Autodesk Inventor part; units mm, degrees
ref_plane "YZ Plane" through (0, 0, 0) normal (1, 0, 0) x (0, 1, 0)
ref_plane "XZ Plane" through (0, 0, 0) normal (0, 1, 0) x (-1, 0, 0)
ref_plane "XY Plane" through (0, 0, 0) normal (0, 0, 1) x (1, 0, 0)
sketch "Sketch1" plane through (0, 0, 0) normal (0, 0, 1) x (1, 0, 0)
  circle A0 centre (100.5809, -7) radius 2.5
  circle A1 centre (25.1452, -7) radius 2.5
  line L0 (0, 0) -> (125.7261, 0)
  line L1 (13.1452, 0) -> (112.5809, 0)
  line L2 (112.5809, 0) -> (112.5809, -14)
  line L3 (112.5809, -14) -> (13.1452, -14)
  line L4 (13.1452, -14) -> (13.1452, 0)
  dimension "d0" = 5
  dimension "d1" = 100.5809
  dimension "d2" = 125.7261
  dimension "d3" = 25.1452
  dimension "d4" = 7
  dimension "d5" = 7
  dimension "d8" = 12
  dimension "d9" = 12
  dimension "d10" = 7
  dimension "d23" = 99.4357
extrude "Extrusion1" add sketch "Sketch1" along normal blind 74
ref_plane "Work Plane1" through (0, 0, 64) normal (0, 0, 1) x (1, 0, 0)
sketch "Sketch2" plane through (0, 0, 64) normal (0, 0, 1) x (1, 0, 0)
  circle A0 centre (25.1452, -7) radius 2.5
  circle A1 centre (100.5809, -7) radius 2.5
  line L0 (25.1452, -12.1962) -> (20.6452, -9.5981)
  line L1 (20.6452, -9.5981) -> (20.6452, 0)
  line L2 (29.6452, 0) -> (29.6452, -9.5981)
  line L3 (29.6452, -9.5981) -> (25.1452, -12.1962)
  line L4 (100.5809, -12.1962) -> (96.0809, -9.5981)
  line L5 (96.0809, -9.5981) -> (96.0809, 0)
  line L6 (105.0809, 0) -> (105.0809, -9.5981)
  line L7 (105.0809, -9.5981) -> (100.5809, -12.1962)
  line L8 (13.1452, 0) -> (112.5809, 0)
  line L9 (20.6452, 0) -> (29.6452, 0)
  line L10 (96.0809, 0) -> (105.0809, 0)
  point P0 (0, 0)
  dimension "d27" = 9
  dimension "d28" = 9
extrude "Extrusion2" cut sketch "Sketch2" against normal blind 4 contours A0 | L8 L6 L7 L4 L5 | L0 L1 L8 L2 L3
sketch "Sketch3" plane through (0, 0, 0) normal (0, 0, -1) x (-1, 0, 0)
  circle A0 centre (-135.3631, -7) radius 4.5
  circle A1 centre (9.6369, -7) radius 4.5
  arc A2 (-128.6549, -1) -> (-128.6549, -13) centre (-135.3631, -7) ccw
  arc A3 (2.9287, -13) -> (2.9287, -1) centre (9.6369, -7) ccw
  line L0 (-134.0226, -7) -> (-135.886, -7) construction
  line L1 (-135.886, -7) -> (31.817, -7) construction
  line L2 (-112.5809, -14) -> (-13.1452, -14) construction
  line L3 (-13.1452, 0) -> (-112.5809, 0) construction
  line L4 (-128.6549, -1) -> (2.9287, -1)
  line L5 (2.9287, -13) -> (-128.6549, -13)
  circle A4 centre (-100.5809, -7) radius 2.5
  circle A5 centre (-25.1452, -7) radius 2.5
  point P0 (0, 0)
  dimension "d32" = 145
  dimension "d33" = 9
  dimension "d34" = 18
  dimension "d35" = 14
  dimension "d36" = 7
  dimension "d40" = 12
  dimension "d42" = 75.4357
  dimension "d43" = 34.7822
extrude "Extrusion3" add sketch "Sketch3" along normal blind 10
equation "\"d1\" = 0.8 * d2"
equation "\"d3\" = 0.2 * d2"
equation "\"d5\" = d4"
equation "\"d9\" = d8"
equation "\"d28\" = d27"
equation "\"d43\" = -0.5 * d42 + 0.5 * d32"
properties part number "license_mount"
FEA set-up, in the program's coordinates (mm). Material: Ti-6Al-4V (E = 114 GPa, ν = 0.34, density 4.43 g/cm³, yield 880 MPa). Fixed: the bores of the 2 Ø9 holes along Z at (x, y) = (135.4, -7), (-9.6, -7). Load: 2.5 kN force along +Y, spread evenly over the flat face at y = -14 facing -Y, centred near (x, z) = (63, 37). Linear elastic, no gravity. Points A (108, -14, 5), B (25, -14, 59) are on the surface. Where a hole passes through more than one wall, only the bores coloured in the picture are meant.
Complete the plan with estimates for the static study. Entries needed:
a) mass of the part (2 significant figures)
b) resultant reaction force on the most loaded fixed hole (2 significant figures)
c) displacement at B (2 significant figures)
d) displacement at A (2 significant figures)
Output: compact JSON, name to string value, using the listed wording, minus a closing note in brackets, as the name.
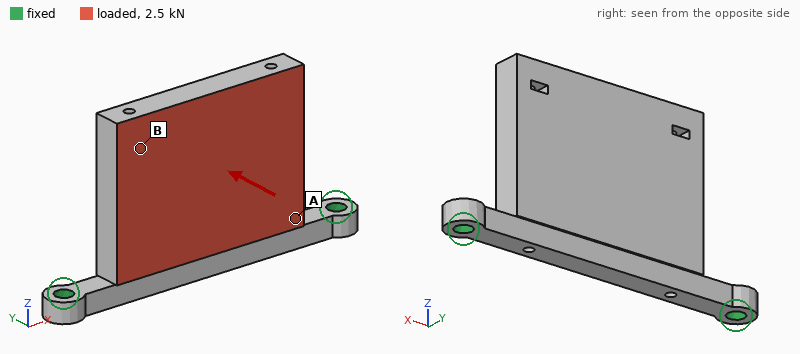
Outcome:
{"mass of the part": "520 g", "resultant reaction force on the most loaded fixed hole": "1.3 kN", "displacement at B": "1.0 mm", "displacement at A": "0.19 mm"}
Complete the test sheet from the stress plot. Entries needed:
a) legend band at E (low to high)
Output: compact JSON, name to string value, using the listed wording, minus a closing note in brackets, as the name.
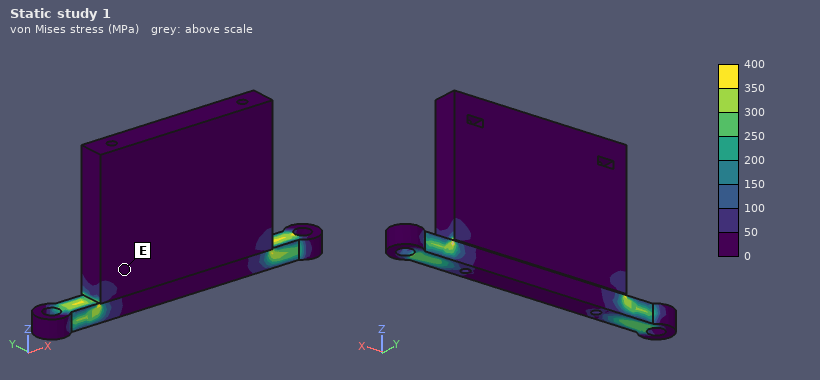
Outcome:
{"legend band at E": "0 to 50 MPa"}
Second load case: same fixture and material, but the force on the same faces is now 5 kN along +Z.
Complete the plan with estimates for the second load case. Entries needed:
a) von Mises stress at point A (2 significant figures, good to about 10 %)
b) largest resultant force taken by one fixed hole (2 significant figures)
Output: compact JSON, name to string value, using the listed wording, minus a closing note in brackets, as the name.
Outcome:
{"von Mises stress at point A": "54 MPa", "largest resultant force taken by one fixed hole": "2.9 kN"}
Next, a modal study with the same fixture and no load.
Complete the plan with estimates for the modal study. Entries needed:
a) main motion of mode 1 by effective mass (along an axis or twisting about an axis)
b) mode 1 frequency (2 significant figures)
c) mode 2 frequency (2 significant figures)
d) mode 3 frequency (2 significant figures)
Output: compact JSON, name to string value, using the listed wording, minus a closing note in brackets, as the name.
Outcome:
{"main motion of mode 1 by effective mass": "along Y", "mode 1 frequency": "420 Hz", "mode 2 frequency": "2500 Hz", "mode 3 frequency": "2500 Hz"}
